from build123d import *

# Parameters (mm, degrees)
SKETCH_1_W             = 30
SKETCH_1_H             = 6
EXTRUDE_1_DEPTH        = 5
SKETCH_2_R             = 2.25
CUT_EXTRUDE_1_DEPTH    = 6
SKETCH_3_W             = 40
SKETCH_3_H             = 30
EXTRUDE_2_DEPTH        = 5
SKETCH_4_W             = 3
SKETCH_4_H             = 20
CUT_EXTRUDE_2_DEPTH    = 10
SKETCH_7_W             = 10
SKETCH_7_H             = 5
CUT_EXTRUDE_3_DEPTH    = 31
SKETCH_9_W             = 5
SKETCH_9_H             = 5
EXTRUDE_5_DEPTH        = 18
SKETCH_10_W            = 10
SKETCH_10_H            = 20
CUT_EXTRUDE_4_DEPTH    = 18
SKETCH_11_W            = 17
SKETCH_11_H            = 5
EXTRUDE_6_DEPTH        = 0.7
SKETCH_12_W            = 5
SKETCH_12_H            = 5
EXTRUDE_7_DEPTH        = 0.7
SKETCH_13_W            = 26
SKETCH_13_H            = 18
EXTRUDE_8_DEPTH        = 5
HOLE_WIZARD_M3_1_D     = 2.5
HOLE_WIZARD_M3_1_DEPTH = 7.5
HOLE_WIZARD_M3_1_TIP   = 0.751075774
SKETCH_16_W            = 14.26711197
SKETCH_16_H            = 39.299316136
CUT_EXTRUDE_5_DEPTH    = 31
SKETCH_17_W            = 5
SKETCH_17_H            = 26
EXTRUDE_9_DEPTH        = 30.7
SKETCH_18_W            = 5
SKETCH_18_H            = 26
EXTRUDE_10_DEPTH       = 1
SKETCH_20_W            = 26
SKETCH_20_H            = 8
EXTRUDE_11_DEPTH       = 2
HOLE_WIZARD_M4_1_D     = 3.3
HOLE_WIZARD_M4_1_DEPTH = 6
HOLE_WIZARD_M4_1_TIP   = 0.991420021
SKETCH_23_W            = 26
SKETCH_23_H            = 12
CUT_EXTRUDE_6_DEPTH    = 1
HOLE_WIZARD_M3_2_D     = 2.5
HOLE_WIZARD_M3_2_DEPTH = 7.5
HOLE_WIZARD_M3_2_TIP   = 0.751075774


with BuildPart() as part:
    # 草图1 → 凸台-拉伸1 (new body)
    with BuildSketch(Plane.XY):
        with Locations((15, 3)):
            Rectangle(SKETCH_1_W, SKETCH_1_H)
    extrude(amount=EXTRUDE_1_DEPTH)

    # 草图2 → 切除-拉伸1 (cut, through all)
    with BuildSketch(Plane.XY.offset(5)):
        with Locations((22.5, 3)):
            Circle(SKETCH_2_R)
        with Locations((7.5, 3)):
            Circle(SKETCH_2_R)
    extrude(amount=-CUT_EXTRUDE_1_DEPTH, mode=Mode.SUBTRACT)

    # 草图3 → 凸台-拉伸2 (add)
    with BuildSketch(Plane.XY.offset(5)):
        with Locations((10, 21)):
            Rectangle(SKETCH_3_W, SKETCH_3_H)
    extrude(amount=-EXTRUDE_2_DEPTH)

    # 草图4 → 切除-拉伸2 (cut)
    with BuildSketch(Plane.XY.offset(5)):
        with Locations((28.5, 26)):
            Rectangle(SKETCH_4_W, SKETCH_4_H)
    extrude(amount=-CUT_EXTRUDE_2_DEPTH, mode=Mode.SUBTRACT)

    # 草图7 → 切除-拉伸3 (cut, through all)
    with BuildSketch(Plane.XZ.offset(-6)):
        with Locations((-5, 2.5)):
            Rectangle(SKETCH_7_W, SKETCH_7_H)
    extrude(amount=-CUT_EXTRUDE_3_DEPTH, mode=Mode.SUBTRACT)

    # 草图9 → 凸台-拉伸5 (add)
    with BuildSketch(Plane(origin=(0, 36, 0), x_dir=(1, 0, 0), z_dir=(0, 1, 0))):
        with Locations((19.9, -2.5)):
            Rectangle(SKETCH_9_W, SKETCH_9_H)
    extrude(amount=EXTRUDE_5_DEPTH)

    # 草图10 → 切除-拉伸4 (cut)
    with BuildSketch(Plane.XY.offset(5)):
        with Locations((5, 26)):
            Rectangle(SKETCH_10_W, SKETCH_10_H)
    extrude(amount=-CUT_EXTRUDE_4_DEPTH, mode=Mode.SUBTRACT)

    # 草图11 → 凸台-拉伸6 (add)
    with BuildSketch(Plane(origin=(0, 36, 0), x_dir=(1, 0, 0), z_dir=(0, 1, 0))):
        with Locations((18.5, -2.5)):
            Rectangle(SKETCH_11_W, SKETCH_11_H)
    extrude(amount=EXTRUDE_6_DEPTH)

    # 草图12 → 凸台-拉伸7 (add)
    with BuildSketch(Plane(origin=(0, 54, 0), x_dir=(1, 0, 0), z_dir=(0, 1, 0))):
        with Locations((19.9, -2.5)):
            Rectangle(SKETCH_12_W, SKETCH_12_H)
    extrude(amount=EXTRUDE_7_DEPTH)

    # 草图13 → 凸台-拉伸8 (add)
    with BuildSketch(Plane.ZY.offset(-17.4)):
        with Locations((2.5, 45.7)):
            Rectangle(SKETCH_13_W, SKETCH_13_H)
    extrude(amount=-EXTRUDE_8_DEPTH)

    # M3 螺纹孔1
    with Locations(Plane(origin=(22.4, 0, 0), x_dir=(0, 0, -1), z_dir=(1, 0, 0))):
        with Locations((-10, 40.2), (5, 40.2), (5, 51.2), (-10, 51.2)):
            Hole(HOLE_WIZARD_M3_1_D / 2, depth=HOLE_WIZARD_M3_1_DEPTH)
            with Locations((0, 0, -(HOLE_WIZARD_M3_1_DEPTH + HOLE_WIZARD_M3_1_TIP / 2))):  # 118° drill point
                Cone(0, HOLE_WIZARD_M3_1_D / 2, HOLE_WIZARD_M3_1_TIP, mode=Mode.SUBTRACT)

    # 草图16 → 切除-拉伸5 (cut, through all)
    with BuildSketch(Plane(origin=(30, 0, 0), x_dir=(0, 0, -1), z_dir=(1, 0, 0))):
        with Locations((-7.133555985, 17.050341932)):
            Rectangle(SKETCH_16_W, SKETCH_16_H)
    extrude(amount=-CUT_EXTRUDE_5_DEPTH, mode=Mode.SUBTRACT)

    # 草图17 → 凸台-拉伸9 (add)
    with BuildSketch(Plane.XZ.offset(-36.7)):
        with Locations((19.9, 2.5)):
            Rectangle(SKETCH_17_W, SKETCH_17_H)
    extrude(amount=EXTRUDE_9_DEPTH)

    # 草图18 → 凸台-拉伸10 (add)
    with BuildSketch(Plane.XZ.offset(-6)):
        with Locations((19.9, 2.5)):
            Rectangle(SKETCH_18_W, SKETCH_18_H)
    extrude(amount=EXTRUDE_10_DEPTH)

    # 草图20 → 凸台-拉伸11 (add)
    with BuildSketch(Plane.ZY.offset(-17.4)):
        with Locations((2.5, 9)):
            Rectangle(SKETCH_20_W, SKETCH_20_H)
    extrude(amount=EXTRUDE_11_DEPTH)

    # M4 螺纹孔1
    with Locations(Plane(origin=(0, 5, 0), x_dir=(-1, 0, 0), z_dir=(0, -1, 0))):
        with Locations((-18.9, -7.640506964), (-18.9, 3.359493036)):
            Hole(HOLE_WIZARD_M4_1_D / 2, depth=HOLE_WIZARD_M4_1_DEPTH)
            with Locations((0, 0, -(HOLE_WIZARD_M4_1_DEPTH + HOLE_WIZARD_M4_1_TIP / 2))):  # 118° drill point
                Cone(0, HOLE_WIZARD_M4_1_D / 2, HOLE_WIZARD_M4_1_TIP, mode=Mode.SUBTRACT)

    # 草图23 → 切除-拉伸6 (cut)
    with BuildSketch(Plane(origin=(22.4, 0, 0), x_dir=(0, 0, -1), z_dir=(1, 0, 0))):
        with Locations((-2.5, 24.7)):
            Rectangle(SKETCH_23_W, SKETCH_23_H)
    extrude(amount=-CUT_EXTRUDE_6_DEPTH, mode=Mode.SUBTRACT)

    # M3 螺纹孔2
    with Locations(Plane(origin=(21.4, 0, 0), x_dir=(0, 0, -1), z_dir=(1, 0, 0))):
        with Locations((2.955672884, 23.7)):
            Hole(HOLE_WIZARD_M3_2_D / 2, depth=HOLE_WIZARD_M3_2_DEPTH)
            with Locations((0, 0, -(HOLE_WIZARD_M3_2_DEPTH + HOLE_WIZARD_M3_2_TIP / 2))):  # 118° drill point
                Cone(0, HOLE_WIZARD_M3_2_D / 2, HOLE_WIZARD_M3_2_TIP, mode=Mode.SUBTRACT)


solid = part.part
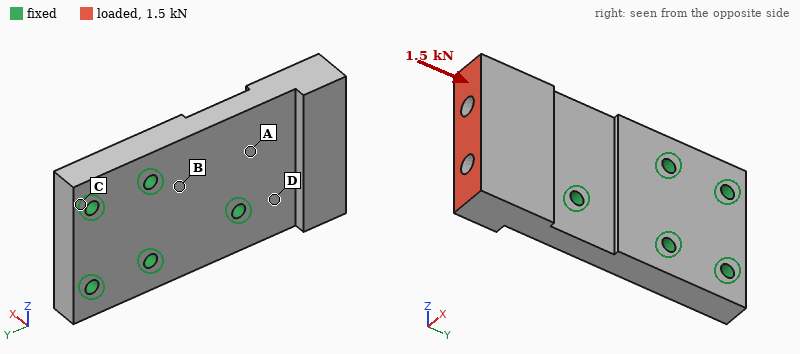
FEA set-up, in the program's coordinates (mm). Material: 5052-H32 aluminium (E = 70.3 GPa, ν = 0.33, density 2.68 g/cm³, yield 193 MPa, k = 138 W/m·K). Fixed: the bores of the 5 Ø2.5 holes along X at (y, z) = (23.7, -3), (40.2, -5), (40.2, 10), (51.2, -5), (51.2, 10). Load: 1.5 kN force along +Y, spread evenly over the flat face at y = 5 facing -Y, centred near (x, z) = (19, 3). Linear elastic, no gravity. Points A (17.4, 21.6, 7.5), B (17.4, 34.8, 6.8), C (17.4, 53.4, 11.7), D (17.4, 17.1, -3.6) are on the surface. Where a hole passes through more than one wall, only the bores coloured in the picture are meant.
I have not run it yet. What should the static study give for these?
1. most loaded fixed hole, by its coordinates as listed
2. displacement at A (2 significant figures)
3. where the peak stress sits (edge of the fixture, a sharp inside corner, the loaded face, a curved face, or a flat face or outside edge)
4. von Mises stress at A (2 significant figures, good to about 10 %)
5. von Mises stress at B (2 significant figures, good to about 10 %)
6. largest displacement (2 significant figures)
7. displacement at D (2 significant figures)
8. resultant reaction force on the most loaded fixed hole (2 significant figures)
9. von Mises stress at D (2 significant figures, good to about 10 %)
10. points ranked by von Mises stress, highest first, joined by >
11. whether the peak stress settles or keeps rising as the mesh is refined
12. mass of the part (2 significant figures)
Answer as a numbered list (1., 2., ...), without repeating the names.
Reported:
1. (23.7, -3)
2. 4.3 µm
3. edge of the fixture
4. 20 MPa
5. 9.8 MPa
6. 21 µm
7. 4.0 µm
8. 790 N
9. 28 MPa
10. D > A > B > C
11. keeps rising
12. 17 g
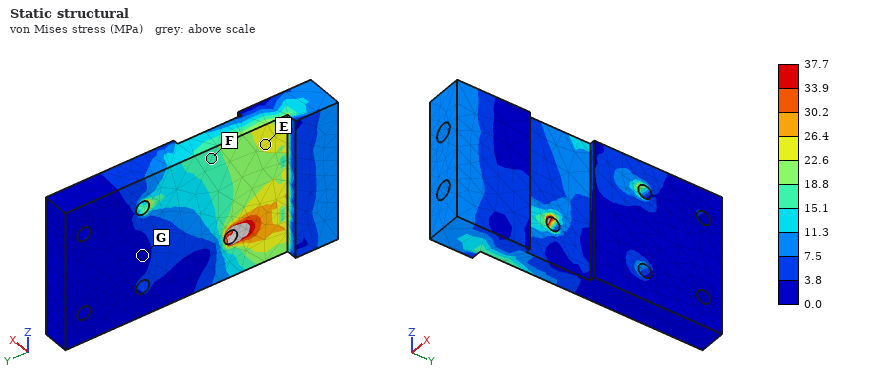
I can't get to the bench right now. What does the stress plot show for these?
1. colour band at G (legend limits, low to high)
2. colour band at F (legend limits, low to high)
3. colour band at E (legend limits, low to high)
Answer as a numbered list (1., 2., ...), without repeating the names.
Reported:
1. 0.0 to 3.8 MPa
2. 15.1 to 18.8 MPa
3. 22.6 to 26.4 MPa
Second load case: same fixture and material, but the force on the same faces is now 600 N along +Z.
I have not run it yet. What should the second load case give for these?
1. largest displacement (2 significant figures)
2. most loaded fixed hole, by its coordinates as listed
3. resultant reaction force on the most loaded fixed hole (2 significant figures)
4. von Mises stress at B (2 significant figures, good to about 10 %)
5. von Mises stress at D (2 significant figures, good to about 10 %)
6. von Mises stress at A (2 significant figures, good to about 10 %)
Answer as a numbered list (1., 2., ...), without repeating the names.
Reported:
1. 17 µm
2. (23.7, -3)
3. 880 N
4. 7.4 MPa
5. 16 MPa
6. 14 MPa
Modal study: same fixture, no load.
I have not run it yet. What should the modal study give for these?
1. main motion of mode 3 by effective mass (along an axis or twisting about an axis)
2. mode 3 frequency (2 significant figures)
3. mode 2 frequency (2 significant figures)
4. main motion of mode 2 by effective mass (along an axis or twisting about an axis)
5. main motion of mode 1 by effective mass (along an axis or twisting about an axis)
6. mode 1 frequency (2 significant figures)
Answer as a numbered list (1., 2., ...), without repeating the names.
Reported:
1. along Z
2. 18 kHz
3. 11 kHz
4. twisting about Y
5. along X
6. 5700 Hz
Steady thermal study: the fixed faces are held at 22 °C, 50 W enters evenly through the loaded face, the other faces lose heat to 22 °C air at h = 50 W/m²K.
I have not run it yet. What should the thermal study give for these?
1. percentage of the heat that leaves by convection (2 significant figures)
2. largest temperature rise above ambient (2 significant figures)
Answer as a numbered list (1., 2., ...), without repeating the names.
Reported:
1. 6.8 %
2. 66 K
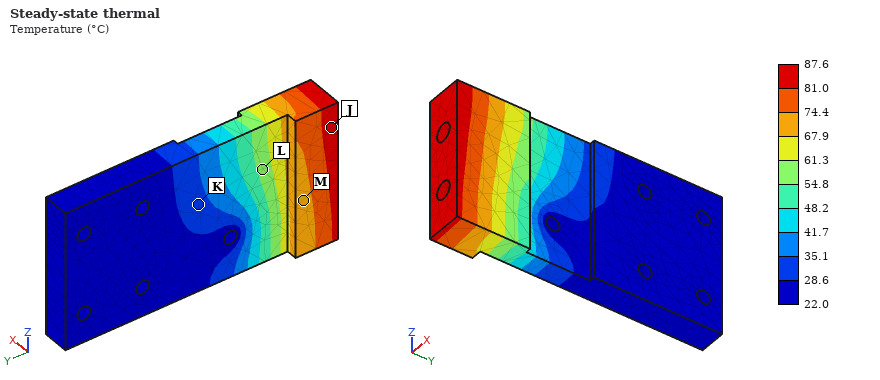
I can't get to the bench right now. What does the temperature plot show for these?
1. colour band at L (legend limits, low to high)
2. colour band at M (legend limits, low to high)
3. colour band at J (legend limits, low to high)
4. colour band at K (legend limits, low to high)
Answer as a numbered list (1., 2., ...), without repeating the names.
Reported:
1. 54.8 to 61.3 °C
2. 67.9 to 74.4 °C
3. 81.0 to 87.6 °C
4. 28.6 to 35.1 °C
